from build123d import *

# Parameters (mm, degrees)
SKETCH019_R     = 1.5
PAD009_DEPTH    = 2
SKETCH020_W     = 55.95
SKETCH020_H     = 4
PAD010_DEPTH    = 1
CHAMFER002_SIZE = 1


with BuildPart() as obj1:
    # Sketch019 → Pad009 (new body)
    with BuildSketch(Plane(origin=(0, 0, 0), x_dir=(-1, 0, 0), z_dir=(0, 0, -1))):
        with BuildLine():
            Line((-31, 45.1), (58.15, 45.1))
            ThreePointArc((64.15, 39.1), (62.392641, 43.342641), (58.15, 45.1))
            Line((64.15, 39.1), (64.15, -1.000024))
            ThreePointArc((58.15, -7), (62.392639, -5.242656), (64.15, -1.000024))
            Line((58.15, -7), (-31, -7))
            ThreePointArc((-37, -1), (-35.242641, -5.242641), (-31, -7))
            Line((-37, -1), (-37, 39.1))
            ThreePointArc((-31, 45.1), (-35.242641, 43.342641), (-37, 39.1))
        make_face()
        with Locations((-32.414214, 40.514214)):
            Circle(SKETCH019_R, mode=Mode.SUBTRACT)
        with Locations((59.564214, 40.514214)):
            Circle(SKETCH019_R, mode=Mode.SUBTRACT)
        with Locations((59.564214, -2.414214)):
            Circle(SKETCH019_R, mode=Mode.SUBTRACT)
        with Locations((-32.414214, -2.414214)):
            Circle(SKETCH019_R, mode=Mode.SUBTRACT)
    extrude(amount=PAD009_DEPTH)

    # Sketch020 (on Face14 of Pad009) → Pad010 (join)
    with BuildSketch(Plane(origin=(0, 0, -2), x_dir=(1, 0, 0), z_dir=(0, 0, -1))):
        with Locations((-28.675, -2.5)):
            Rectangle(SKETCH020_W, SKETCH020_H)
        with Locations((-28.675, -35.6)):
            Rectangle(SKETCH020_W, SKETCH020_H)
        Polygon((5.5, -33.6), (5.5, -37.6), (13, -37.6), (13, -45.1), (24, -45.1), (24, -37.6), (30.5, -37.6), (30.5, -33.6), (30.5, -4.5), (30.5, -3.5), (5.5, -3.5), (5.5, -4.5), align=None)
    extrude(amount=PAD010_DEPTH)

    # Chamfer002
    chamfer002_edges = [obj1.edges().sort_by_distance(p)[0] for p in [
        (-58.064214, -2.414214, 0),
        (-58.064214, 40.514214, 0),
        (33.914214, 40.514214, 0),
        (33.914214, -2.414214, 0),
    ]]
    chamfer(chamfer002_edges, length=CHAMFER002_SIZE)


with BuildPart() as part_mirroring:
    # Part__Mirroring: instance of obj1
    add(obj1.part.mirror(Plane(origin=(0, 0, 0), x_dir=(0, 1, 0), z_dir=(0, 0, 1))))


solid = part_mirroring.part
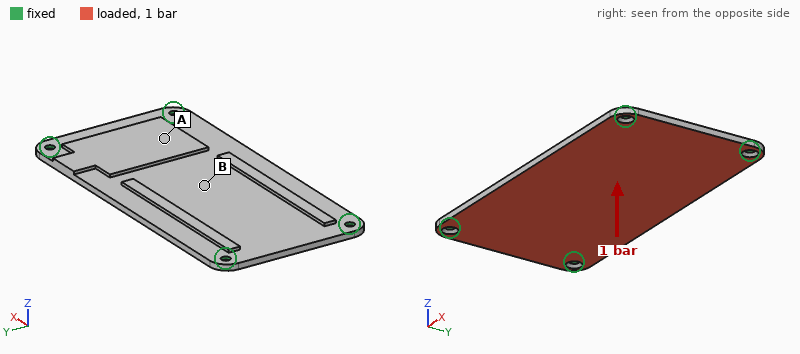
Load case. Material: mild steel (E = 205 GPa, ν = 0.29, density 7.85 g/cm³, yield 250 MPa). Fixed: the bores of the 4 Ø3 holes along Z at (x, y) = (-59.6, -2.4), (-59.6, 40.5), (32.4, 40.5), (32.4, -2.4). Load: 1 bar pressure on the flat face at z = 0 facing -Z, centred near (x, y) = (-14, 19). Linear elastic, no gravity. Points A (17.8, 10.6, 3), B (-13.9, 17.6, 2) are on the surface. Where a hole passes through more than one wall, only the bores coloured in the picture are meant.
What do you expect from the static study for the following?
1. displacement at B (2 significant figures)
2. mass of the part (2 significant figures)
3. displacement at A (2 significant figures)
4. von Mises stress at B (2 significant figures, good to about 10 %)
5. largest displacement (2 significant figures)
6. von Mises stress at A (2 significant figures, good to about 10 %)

0.17 mm
92 g
0.070 mm
41 MPa
0.17 mm
17 MPa
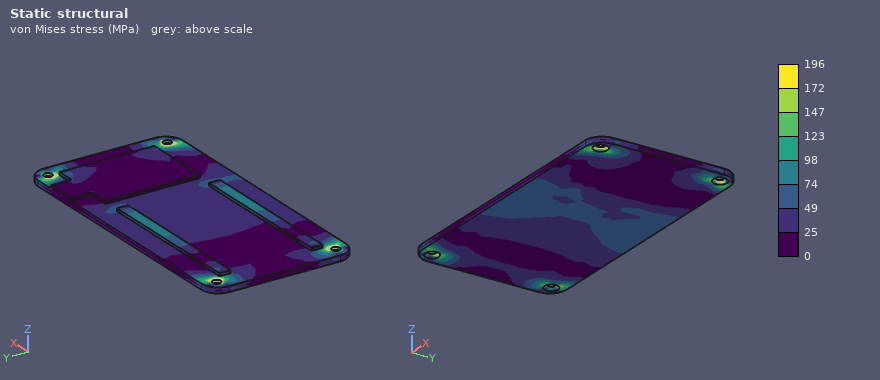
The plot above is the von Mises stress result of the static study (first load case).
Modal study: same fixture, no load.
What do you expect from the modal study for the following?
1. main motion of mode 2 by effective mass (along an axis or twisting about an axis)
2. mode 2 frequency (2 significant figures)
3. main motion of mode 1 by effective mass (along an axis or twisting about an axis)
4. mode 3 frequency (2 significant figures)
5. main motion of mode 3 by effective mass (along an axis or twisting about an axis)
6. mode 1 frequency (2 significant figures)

twisting about X
2100 Hz
along Z
3000 Hz
twisting about Y
1100 Hz
